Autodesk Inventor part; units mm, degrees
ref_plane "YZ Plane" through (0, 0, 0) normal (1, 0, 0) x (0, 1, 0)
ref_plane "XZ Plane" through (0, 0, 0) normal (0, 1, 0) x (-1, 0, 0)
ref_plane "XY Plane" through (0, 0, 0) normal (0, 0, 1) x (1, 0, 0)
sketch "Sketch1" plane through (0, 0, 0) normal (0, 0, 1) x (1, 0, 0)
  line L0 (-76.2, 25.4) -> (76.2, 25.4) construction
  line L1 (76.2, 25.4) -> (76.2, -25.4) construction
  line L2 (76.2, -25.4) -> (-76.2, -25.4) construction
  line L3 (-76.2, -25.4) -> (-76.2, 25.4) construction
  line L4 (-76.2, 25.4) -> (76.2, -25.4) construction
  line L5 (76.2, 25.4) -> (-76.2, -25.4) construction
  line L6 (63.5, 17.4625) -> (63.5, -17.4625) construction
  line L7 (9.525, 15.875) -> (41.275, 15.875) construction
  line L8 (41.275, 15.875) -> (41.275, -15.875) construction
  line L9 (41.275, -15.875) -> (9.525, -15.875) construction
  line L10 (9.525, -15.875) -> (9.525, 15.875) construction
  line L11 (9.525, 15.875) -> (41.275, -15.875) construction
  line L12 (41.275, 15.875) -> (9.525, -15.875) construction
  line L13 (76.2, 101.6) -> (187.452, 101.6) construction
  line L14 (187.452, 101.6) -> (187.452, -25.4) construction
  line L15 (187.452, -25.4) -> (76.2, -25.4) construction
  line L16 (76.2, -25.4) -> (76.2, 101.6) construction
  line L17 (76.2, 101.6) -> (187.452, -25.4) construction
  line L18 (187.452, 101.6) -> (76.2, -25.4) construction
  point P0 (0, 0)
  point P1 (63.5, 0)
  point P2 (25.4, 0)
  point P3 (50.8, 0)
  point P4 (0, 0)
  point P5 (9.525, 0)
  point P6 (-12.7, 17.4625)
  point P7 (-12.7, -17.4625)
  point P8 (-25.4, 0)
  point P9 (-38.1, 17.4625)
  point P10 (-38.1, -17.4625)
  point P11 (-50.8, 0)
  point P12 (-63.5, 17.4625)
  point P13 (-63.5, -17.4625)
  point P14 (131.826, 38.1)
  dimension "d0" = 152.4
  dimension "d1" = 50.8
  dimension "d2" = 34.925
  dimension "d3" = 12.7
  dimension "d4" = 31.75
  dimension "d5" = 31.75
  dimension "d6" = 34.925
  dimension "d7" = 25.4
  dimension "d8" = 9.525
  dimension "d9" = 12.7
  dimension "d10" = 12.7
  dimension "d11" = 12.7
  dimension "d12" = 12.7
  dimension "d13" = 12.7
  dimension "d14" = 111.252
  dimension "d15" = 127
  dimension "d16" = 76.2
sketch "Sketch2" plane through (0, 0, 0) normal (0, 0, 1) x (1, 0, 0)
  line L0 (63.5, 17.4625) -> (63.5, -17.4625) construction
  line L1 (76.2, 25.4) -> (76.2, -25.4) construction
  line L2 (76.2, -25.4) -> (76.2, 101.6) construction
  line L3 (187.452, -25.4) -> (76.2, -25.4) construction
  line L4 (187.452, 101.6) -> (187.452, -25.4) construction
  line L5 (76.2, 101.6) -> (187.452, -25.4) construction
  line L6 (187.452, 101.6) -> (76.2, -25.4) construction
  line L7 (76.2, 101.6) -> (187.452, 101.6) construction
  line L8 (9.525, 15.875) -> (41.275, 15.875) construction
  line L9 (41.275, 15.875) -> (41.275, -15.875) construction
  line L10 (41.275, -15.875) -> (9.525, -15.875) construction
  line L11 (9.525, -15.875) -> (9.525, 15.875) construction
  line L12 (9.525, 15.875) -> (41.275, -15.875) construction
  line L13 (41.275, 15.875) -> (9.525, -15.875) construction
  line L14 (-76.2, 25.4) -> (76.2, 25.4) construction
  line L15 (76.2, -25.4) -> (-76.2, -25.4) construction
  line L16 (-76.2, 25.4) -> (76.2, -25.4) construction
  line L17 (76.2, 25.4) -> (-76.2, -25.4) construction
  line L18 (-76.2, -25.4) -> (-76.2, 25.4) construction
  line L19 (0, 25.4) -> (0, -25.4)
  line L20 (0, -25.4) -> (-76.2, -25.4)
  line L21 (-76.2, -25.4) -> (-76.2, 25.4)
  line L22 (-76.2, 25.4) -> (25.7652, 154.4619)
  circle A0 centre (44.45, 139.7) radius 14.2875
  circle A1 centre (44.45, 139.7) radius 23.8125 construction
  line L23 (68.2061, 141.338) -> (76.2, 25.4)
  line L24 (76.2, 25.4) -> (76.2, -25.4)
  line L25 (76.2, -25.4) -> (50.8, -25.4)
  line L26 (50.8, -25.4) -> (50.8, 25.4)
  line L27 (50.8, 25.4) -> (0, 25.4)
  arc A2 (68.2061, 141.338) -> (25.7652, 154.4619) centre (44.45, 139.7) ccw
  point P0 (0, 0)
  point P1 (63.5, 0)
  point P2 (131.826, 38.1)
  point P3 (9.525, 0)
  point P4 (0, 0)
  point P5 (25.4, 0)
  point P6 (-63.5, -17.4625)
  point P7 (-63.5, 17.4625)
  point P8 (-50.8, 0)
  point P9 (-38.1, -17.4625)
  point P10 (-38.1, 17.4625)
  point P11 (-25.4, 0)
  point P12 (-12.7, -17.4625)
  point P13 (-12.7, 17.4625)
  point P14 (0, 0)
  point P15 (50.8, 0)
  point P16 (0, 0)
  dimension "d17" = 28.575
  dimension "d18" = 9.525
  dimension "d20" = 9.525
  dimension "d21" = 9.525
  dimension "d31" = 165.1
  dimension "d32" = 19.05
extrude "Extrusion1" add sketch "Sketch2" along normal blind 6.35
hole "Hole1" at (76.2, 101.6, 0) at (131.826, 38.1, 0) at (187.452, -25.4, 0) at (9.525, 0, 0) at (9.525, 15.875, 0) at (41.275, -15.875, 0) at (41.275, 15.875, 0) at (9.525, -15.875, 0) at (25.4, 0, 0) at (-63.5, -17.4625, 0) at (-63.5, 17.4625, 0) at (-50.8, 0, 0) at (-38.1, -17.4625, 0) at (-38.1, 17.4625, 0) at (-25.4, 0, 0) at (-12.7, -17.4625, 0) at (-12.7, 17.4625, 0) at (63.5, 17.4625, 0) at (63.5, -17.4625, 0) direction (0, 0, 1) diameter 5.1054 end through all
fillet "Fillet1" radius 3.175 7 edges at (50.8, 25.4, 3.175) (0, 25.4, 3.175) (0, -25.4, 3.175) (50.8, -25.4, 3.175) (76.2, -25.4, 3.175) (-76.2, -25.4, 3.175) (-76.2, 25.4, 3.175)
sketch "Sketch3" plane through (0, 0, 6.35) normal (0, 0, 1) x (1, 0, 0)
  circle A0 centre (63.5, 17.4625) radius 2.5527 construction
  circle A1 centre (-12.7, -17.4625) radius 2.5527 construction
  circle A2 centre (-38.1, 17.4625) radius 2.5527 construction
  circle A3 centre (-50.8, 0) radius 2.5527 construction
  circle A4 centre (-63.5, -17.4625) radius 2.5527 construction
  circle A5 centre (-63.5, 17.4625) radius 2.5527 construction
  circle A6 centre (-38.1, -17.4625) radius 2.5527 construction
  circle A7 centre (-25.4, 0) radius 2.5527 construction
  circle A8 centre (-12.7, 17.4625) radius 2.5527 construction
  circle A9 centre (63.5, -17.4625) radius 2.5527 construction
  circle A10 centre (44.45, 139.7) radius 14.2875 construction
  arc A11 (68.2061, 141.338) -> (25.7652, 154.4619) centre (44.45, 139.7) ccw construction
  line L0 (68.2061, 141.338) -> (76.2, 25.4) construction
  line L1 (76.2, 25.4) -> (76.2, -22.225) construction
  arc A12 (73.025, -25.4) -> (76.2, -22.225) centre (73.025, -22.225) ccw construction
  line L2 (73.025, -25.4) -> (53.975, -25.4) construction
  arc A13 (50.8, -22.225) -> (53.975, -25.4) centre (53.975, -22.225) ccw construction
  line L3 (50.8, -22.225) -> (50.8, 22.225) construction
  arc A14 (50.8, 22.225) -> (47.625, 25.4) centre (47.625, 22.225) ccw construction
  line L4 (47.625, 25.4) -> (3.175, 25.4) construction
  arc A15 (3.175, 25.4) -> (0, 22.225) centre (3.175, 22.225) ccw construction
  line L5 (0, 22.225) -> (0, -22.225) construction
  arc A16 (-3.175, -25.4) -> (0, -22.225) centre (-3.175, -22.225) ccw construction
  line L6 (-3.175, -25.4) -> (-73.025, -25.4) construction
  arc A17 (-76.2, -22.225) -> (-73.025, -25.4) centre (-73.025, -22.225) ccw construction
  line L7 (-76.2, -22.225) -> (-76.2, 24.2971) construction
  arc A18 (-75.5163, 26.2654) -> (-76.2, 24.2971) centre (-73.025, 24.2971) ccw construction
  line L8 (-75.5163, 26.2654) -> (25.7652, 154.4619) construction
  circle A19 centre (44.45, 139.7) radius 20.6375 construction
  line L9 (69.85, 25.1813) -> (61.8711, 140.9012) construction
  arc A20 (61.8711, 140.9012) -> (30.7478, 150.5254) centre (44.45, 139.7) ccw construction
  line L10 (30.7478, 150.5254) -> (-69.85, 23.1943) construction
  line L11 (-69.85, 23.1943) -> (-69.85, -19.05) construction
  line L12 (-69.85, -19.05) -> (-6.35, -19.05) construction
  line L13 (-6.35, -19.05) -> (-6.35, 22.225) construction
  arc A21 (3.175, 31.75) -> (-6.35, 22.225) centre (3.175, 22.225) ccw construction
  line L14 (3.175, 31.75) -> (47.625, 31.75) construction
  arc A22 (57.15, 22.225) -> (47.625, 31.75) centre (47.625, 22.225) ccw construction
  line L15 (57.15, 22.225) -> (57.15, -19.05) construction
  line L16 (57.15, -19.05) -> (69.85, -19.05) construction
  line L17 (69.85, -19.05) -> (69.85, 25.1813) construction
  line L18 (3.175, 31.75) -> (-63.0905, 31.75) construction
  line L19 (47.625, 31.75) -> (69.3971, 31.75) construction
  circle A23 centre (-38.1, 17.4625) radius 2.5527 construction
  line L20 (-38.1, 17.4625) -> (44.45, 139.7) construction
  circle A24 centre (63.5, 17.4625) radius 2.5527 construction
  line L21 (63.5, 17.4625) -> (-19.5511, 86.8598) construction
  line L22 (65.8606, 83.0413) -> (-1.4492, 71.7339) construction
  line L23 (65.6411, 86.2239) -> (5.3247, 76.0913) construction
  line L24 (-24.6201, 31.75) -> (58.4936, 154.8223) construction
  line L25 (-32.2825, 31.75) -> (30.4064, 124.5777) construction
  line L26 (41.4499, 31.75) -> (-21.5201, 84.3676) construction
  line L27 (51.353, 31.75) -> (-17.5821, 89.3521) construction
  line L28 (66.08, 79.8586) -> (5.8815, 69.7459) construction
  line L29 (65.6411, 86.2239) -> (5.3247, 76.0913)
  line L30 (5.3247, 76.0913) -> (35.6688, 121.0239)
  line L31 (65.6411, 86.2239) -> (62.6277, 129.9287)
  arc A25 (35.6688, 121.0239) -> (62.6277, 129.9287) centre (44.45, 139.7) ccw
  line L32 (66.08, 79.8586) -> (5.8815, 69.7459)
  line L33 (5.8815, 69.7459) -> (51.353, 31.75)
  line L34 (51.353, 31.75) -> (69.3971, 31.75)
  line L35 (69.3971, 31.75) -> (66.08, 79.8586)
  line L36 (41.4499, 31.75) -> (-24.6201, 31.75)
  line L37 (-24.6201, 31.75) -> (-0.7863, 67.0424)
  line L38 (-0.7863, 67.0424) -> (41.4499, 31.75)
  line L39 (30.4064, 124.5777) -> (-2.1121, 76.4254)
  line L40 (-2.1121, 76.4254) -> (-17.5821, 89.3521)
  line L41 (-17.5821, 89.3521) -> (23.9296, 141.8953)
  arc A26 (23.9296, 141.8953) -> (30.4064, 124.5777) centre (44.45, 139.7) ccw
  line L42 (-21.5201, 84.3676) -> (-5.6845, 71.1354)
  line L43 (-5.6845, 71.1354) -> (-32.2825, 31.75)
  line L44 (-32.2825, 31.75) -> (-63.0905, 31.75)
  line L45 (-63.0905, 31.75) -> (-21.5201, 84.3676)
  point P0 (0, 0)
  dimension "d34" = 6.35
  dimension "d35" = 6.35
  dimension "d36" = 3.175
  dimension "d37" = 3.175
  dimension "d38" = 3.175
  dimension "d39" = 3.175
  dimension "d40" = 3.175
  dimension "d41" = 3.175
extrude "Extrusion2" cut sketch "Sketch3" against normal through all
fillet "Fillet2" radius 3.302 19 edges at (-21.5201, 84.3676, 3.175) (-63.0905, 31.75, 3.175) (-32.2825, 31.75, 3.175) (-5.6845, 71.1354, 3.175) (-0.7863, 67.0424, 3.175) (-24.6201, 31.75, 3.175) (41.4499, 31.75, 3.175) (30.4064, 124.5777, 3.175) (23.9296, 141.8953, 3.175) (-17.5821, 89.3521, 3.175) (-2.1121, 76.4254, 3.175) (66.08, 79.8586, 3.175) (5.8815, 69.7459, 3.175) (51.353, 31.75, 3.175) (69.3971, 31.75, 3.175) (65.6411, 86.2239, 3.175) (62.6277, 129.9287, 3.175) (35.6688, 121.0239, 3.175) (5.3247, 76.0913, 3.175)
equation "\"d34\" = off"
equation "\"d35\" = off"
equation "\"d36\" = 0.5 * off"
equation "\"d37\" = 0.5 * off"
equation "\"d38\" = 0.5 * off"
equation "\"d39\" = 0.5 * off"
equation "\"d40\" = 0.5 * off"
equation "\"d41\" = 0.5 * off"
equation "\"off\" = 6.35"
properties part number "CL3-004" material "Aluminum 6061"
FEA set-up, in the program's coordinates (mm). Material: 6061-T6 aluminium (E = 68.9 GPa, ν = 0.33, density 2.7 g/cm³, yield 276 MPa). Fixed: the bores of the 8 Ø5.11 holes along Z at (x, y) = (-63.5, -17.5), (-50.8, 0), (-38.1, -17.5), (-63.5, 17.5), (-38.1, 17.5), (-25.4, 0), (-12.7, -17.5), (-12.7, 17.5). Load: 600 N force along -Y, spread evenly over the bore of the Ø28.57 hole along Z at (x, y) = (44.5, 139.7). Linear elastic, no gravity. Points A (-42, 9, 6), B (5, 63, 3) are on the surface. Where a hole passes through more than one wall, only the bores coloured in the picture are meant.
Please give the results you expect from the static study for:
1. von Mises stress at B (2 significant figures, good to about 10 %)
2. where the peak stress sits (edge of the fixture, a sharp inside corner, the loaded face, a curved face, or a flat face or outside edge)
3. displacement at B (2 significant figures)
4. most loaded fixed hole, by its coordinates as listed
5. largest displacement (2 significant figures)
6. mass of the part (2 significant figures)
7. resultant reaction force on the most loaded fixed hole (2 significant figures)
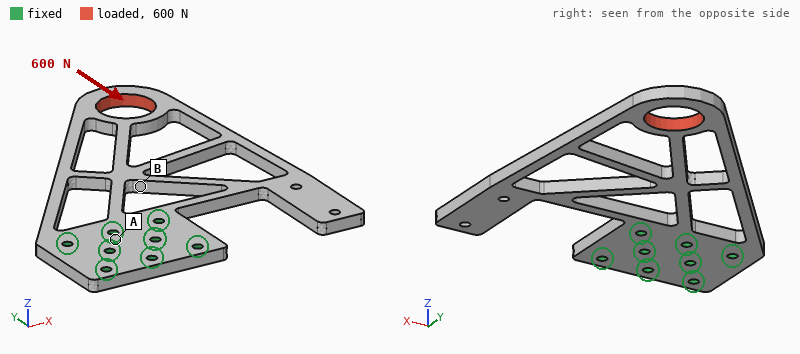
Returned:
23 MPa
a curved face
0.20 mm
(-63.5, 17.5)
0.66 mm
170 g
810 N
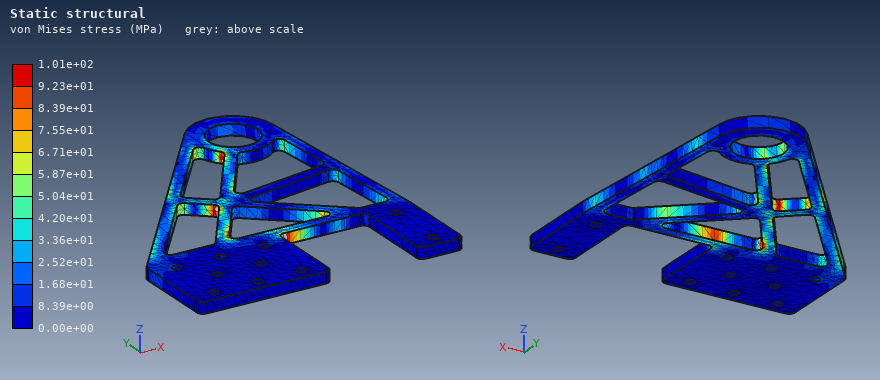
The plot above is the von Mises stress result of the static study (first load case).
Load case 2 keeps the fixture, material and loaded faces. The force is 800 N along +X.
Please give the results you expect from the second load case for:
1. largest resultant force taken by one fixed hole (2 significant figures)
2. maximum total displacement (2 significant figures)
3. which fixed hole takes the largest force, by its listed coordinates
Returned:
1.9 kN
1.1 mm
(-63.5, 17.5)
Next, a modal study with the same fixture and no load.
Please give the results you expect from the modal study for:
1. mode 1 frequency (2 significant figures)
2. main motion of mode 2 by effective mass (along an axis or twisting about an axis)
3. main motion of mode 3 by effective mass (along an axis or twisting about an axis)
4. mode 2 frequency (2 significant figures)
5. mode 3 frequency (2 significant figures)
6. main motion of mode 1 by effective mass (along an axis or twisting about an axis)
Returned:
160 Hz
along Z
along Y
290 Hz
560 Hz
along Z
